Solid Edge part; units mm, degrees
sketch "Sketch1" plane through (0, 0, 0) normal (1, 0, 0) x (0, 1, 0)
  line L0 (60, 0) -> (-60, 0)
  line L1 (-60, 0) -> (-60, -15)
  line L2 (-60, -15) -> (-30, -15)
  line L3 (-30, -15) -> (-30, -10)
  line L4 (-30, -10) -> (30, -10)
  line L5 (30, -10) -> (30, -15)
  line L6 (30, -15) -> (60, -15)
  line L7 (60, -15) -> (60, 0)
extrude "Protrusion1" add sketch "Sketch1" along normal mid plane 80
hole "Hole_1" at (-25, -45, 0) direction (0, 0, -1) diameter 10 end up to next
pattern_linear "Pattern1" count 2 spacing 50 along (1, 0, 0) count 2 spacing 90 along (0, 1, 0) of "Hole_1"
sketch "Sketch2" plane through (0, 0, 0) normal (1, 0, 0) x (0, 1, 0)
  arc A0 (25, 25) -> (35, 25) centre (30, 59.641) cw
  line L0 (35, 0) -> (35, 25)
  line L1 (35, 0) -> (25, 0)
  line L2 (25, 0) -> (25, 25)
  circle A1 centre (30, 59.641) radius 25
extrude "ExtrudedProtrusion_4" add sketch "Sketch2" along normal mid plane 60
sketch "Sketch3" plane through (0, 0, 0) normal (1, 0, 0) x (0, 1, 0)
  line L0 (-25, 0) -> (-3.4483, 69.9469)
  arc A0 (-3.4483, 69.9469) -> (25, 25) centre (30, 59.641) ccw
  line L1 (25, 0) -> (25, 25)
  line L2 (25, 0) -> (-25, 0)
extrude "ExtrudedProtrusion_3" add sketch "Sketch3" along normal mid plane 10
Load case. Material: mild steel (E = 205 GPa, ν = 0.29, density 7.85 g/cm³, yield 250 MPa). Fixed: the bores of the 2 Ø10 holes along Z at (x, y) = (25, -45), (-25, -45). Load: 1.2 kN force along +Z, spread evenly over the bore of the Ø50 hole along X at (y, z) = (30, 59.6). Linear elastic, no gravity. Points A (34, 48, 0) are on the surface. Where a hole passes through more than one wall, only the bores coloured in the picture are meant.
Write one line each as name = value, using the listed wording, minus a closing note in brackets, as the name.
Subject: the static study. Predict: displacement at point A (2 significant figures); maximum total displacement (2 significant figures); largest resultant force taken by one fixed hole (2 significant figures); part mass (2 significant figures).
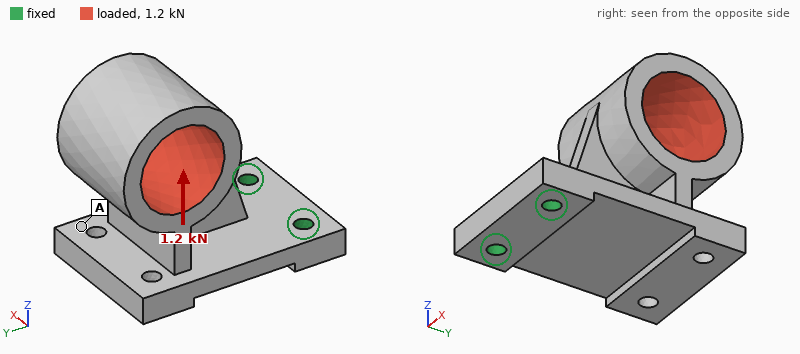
displacement at point A = 0.091 mm
maximum total displacement = 0.15 mm
largest resultant force taken by one fixed hole = 600 N
part mass = 2.0 kg
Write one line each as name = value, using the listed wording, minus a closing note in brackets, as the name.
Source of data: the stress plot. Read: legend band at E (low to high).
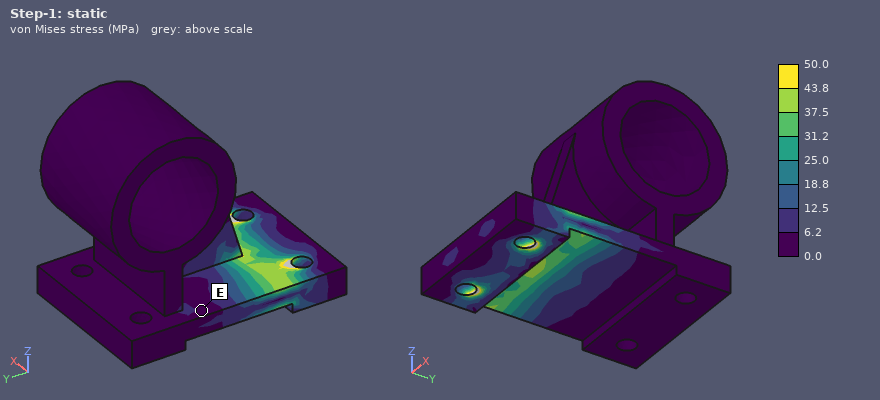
legend band at E = 0.0 to 6.2 MPa
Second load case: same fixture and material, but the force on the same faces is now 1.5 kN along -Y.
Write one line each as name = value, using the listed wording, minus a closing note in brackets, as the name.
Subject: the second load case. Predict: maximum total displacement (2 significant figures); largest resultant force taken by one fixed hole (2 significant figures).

maximum total displacement = 0.22 mm
largest resultant force taken by one fixed hole = 820 N
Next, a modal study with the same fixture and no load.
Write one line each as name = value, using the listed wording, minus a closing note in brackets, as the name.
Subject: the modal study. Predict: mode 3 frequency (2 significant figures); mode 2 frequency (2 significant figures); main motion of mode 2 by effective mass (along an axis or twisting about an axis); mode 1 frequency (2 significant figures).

mode 3 frequency = 2400 Hz
mode 2 frequency = 600 Hz
main motion of mode 2 by effective mass = along X
mode 1 frequency = 380 Hz
